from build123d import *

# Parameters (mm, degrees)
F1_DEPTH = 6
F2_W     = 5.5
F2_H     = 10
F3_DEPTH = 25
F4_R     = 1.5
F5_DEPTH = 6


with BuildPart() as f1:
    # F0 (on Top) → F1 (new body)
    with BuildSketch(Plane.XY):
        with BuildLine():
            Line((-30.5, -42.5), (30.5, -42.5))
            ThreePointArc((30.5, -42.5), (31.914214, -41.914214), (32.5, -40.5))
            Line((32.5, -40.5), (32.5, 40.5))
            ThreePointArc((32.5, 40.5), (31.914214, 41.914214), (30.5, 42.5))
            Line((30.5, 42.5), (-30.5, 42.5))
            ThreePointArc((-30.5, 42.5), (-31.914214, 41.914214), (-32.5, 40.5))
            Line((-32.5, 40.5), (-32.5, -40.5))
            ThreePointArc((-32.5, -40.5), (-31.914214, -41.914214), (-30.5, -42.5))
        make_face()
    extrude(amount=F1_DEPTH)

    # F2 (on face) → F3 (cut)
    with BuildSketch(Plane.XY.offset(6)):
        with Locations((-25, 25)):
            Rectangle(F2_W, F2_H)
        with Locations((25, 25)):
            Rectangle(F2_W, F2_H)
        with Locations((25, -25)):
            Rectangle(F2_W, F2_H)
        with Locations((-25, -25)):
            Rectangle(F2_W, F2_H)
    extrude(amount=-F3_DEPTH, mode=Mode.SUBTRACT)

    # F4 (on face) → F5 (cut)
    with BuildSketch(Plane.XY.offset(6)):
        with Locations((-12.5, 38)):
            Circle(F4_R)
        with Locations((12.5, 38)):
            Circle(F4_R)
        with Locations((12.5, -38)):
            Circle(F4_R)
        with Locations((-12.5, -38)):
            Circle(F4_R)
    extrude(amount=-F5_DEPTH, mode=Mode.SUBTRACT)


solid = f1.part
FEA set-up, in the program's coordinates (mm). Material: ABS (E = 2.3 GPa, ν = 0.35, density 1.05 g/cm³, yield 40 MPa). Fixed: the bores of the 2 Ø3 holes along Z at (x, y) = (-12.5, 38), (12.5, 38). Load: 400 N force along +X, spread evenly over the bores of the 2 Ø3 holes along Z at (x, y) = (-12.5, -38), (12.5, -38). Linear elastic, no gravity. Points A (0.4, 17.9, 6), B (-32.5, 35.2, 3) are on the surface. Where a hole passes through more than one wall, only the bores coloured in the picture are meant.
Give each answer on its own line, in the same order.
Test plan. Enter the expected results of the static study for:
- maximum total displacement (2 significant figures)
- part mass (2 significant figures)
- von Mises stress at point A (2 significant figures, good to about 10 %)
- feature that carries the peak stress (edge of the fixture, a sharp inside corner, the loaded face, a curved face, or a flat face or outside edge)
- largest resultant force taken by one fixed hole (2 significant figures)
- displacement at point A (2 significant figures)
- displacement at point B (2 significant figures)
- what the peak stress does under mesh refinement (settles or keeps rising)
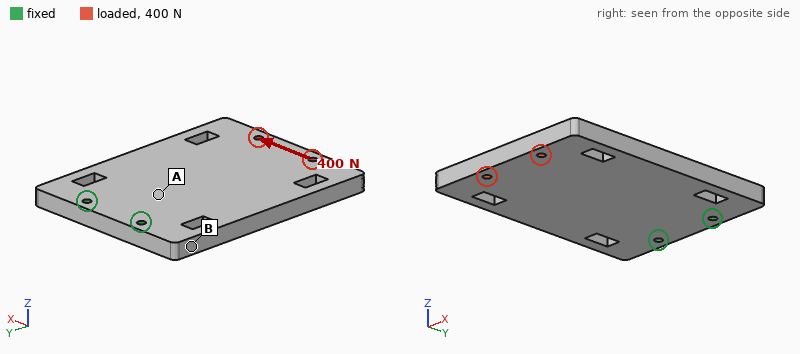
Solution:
0.97 mm
33 g
6.1 MPa
edge of the fixture
1.1 kN
0.18 mm
0.30 mm
keeps rising
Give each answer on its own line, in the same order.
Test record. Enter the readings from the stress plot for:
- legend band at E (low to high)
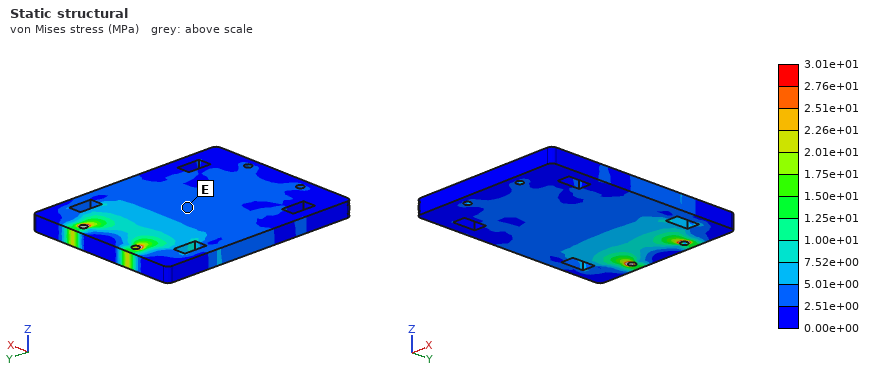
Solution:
2.51e+00 to 5.01e+00 MPa
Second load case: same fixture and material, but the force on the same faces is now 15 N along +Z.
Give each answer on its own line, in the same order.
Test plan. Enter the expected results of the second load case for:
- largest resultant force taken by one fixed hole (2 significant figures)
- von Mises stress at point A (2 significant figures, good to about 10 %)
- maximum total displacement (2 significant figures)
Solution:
7.5 N
2.2 MPa
1.2 mm
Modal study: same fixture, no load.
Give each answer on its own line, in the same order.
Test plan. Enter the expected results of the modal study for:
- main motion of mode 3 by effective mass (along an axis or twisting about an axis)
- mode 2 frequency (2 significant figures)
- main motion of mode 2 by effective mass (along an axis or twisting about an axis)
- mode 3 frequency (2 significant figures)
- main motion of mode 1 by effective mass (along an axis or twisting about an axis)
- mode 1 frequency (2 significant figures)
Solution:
along X
550 Hz
twisting about Y
960 Hz
along Z
200 Hz
